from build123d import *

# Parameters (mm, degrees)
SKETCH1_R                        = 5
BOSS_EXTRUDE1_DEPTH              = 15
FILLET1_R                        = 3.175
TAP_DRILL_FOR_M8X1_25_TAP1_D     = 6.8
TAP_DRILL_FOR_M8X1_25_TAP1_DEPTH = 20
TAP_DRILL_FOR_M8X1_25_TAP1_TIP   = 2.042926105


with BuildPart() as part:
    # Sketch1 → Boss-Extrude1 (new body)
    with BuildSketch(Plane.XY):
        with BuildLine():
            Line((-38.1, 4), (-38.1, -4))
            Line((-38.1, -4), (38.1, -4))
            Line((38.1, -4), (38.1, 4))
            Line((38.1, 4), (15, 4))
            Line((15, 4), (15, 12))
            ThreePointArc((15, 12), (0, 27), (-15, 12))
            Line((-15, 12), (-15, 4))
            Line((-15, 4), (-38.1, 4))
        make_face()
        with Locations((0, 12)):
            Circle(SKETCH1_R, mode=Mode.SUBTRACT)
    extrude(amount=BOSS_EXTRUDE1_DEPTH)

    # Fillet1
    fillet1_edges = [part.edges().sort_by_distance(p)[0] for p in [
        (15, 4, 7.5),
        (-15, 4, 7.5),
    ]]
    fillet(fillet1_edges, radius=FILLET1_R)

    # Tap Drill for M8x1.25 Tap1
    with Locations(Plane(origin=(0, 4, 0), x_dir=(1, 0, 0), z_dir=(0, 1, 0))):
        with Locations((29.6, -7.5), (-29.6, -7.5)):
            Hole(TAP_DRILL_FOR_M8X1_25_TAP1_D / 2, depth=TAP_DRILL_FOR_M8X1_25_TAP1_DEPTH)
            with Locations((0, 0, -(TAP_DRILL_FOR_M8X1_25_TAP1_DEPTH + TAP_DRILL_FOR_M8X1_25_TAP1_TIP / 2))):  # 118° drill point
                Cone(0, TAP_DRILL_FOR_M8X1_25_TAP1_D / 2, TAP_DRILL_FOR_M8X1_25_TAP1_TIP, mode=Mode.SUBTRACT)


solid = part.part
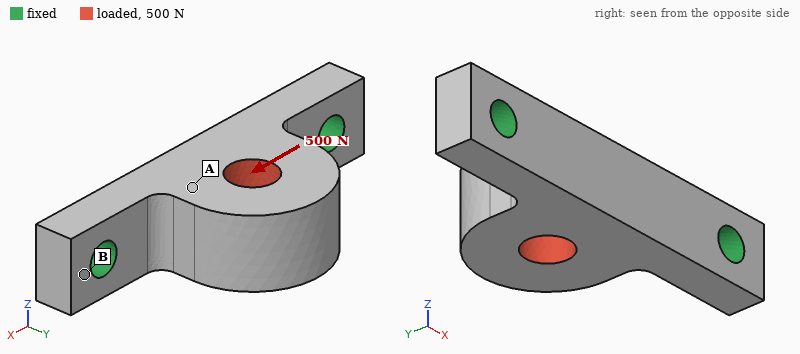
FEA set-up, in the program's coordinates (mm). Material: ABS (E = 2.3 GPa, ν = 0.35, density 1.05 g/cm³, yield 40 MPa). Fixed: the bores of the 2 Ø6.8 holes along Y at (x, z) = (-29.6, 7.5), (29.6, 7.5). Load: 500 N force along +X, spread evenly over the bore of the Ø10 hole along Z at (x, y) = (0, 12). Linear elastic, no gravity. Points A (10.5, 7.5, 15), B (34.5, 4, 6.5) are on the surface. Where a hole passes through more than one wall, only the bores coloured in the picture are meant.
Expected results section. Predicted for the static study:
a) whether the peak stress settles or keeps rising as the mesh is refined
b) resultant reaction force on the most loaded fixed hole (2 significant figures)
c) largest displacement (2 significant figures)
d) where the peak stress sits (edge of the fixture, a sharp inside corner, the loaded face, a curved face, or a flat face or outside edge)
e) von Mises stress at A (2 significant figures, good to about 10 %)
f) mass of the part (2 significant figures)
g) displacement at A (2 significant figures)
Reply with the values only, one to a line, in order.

keeps rising
280 N
83 µm
edge of the fixture
2.7 MPa
17 g
35 µm
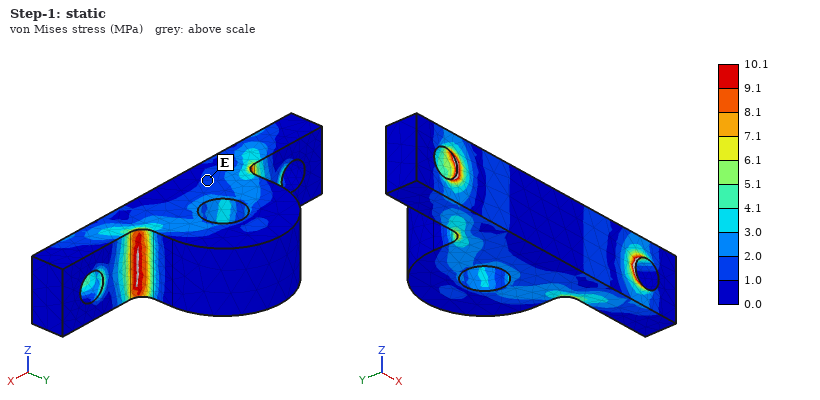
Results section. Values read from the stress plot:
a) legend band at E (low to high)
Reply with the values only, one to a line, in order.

1.0 to 2.0 MPa
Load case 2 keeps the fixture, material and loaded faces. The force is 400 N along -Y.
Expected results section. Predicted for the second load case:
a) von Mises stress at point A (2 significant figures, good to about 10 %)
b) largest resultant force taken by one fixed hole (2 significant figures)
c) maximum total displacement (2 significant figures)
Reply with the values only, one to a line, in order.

2.1 MPa
220 N
96 µm
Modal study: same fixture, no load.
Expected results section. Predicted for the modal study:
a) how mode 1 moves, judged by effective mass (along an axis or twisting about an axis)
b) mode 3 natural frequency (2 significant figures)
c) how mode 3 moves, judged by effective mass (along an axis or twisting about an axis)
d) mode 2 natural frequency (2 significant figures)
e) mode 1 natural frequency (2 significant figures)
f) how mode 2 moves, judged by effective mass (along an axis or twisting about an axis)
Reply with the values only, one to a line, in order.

along Z
4100 Hz
along X
3100 Hz
1400 Hz
along Y
